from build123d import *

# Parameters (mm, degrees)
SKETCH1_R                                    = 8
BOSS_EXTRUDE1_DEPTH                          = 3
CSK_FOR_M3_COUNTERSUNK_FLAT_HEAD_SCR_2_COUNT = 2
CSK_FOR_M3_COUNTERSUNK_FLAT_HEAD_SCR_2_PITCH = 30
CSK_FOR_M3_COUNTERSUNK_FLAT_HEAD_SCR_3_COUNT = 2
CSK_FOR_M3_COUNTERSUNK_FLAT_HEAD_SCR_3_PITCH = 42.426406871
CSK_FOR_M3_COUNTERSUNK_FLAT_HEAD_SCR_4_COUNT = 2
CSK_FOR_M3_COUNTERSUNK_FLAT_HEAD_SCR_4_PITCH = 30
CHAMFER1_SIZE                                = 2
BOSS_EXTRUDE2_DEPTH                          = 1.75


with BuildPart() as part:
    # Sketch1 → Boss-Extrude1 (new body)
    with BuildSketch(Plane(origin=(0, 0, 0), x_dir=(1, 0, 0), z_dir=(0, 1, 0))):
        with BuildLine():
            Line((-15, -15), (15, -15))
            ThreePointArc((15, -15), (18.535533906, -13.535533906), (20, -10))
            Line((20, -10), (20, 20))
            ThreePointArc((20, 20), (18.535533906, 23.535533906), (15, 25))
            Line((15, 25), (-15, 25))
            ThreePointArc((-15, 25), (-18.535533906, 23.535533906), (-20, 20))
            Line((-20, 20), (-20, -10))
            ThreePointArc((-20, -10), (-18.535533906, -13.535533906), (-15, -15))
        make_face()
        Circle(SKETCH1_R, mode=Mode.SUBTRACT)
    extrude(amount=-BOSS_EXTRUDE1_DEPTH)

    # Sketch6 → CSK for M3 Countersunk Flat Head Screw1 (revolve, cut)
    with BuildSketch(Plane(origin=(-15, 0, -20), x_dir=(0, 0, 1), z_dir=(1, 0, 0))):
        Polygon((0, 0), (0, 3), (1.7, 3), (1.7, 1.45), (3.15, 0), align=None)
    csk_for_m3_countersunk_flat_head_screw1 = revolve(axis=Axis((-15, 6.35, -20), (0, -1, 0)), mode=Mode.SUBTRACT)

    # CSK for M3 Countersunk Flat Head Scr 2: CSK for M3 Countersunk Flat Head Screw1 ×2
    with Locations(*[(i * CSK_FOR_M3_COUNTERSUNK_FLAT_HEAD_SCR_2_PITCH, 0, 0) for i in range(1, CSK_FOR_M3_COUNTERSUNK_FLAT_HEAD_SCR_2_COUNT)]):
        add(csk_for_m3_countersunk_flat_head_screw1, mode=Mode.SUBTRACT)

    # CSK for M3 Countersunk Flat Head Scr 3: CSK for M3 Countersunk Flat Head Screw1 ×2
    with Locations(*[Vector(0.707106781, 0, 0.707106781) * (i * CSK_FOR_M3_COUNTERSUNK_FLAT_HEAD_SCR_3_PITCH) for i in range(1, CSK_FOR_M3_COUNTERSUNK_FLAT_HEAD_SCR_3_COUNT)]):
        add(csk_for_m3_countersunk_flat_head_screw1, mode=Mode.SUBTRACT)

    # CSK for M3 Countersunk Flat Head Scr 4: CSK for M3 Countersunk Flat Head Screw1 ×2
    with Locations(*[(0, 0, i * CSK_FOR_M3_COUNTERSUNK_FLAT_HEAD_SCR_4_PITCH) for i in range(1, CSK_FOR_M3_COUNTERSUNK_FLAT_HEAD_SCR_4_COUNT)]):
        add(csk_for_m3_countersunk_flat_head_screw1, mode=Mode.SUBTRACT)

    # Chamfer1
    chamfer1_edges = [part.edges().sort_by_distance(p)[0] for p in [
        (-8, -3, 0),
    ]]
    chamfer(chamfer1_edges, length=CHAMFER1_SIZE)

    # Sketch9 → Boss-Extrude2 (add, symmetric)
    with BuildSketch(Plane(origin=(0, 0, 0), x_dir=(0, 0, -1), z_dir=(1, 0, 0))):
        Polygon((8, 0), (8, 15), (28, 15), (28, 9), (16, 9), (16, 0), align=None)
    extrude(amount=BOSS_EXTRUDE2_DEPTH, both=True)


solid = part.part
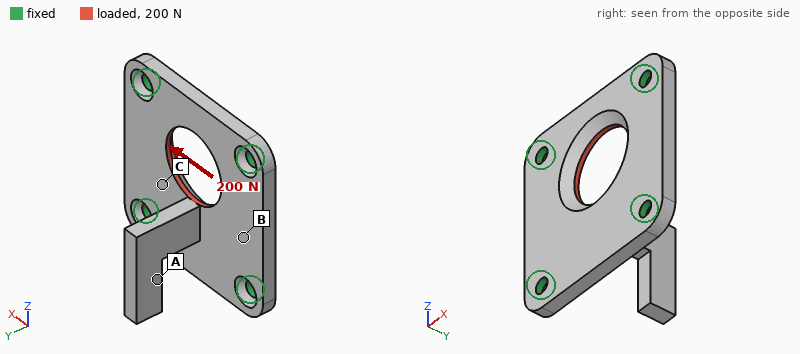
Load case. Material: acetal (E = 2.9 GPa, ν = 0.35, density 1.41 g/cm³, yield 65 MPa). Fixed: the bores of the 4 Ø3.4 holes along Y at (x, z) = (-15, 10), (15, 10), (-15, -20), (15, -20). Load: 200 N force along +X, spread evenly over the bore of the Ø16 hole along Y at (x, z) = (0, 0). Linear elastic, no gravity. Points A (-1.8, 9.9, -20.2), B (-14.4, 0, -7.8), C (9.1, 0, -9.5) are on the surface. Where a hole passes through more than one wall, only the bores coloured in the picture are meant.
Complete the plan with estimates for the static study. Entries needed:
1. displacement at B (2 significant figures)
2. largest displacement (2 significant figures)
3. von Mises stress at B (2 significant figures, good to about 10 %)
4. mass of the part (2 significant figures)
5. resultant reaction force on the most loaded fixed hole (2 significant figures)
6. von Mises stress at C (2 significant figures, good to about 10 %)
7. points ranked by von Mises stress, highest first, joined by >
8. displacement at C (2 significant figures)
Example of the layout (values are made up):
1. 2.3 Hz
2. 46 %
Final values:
1. 13 µm
2. 25 µm
3. 1.5 MPa
4. 6.4 g
5. 60 N
6. 2.2 MPa
7. C > B > A
8. 11 µm
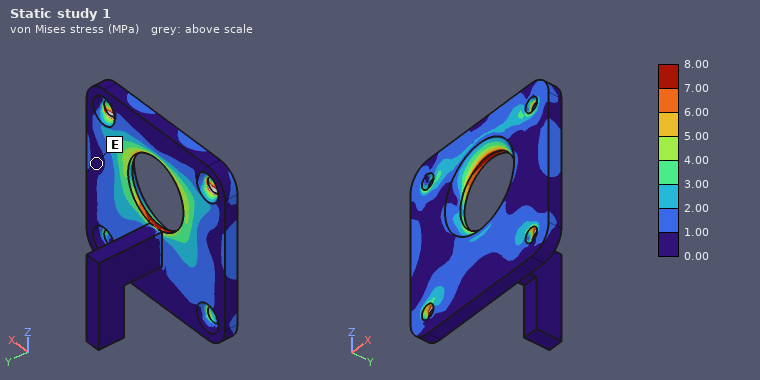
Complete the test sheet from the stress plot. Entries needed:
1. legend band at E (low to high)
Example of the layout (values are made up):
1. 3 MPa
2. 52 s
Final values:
1. 0.00 to 1.00 MPa
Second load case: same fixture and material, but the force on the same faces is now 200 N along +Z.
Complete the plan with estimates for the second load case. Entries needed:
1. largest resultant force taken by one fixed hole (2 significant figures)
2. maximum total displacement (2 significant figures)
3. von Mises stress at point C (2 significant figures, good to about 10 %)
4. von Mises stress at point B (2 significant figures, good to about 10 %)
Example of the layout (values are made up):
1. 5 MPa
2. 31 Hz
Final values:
1. 55 N
2. 37 µm
3. 2.1 MPa
4. 1.4 MPa
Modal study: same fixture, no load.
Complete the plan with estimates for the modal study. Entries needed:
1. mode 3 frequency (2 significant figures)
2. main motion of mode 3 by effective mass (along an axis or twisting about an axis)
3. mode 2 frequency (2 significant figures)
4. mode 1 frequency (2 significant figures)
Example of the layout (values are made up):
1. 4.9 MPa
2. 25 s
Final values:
1. 2500 Hz
2. along Y
3. 1700 Hz
4. 1400 Hz
